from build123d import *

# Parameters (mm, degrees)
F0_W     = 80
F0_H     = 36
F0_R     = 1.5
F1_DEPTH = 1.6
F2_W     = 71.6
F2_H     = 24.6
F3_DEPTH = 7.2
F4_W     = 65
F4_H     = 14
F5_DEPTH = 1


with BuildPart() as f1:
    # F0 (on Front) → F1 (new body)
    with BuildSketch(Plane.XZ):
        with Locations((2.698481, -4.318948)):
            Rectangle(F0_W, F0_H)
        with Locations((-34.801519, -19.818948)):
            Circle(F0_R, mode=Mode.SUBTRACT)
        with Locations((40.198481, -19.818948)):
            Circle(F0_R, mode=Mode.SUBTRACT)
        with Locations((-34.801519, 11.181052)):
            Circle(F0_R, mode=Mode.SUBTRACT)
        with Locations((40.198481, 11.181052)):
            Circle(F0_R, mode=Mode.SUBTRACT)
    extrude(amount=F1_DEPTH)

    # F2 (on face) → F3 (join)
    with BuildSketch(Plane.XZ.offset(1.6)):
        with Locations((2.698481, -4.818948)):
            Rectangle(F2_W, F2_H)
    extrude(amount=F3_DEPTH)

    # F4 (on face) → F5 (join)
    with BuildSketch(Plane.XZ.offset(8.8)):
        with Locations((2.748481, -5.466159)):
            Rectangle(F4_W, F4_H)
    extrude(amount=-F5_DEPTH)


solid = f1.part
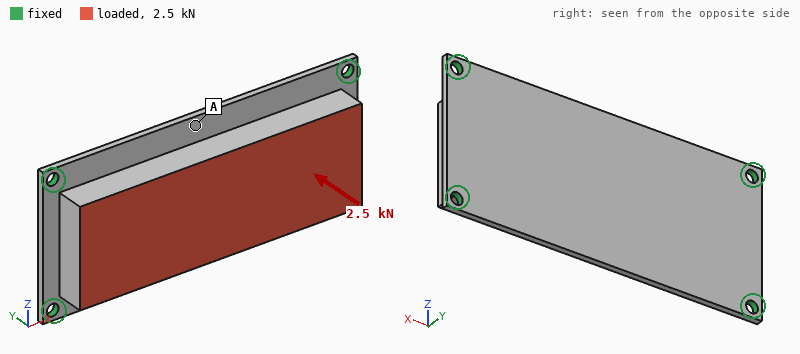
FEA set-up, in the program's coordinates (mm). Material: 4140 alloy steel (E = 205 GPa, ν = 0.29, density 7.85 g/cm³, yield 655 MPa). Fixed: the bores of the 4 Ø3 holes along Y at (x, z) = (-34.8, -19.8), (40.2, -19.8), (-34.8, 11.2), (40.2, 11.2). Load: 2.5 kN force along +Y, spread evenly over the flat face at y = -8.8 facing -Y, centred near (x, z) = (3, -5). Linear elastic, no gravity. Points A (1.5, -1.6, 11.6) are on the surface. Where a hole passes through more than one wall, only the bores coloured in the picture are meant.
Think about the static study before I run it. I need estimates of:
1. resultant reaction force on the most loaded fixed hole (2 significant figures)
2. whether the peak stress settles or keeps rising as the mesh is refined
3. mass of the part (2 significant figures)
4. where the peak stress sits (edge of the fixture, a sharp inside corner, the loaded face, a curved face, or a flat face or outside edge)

1.2 kN
keeps rising
140 g
edge of the fixture
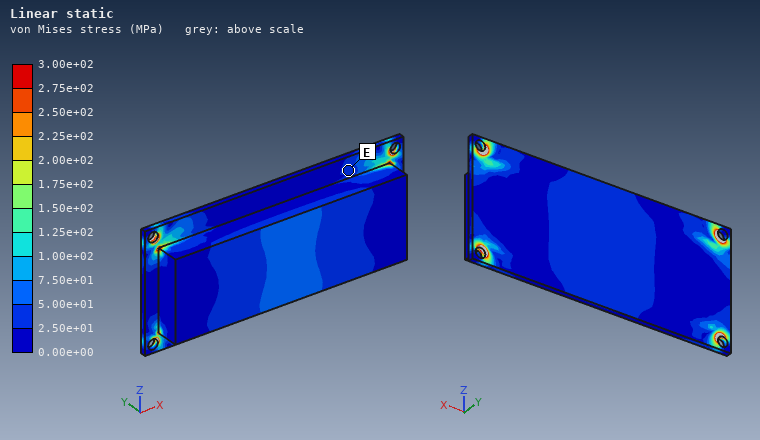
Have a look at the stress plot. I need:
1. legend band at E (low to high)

2.50e+01 to 5.00e+01 MPa
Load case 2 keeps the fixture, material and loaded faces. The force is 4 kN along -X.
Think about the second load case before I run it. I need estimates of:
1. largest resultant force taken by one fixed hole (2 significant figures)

1.2 kN
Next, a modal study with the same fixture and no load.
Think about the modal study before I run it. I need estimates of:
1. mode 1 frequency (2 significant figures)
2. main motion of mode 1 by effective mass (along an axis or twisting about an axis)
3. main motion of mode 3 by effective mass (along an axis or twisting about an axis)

3900 Hz
along Y
twisting about Z
